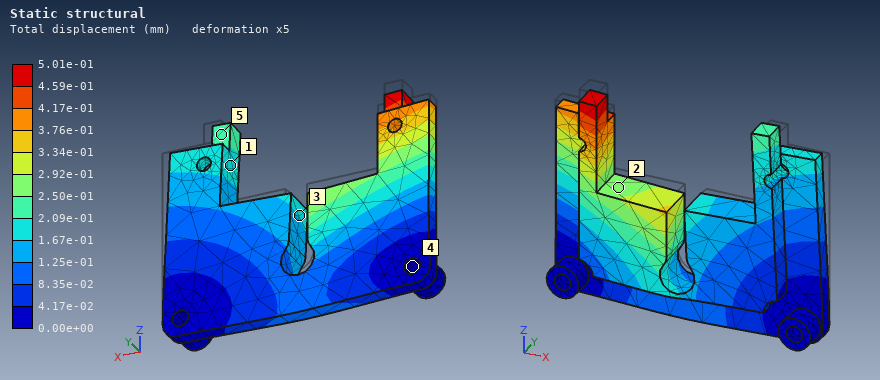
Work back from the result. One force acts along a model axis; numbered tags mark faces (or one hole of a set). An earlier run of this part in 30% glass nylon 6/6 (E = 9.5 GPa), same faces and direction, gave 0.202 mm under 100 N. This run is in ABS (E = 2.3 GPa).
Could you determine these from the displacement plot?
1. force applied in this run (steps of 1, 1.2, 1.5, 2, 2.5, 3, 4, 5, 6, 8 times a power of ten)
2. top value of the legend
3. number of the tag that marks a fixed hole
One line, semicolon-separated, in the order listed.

60 N; 5.01e-01 mm; 4
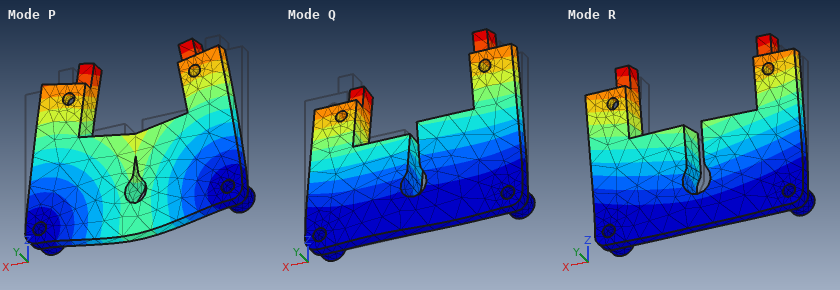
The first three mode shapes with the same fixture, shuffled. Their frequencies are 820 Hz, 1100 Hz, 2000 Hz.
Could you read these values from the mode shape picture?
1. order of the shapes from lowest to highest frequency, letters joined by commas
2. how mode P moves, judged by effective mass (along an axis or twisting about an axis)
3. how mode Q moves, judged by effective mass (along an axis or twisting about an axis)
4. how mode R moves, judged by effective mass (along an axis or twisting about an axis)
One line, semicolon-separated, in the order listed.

R, Q, P; along Z; twisting about Z; along Y
